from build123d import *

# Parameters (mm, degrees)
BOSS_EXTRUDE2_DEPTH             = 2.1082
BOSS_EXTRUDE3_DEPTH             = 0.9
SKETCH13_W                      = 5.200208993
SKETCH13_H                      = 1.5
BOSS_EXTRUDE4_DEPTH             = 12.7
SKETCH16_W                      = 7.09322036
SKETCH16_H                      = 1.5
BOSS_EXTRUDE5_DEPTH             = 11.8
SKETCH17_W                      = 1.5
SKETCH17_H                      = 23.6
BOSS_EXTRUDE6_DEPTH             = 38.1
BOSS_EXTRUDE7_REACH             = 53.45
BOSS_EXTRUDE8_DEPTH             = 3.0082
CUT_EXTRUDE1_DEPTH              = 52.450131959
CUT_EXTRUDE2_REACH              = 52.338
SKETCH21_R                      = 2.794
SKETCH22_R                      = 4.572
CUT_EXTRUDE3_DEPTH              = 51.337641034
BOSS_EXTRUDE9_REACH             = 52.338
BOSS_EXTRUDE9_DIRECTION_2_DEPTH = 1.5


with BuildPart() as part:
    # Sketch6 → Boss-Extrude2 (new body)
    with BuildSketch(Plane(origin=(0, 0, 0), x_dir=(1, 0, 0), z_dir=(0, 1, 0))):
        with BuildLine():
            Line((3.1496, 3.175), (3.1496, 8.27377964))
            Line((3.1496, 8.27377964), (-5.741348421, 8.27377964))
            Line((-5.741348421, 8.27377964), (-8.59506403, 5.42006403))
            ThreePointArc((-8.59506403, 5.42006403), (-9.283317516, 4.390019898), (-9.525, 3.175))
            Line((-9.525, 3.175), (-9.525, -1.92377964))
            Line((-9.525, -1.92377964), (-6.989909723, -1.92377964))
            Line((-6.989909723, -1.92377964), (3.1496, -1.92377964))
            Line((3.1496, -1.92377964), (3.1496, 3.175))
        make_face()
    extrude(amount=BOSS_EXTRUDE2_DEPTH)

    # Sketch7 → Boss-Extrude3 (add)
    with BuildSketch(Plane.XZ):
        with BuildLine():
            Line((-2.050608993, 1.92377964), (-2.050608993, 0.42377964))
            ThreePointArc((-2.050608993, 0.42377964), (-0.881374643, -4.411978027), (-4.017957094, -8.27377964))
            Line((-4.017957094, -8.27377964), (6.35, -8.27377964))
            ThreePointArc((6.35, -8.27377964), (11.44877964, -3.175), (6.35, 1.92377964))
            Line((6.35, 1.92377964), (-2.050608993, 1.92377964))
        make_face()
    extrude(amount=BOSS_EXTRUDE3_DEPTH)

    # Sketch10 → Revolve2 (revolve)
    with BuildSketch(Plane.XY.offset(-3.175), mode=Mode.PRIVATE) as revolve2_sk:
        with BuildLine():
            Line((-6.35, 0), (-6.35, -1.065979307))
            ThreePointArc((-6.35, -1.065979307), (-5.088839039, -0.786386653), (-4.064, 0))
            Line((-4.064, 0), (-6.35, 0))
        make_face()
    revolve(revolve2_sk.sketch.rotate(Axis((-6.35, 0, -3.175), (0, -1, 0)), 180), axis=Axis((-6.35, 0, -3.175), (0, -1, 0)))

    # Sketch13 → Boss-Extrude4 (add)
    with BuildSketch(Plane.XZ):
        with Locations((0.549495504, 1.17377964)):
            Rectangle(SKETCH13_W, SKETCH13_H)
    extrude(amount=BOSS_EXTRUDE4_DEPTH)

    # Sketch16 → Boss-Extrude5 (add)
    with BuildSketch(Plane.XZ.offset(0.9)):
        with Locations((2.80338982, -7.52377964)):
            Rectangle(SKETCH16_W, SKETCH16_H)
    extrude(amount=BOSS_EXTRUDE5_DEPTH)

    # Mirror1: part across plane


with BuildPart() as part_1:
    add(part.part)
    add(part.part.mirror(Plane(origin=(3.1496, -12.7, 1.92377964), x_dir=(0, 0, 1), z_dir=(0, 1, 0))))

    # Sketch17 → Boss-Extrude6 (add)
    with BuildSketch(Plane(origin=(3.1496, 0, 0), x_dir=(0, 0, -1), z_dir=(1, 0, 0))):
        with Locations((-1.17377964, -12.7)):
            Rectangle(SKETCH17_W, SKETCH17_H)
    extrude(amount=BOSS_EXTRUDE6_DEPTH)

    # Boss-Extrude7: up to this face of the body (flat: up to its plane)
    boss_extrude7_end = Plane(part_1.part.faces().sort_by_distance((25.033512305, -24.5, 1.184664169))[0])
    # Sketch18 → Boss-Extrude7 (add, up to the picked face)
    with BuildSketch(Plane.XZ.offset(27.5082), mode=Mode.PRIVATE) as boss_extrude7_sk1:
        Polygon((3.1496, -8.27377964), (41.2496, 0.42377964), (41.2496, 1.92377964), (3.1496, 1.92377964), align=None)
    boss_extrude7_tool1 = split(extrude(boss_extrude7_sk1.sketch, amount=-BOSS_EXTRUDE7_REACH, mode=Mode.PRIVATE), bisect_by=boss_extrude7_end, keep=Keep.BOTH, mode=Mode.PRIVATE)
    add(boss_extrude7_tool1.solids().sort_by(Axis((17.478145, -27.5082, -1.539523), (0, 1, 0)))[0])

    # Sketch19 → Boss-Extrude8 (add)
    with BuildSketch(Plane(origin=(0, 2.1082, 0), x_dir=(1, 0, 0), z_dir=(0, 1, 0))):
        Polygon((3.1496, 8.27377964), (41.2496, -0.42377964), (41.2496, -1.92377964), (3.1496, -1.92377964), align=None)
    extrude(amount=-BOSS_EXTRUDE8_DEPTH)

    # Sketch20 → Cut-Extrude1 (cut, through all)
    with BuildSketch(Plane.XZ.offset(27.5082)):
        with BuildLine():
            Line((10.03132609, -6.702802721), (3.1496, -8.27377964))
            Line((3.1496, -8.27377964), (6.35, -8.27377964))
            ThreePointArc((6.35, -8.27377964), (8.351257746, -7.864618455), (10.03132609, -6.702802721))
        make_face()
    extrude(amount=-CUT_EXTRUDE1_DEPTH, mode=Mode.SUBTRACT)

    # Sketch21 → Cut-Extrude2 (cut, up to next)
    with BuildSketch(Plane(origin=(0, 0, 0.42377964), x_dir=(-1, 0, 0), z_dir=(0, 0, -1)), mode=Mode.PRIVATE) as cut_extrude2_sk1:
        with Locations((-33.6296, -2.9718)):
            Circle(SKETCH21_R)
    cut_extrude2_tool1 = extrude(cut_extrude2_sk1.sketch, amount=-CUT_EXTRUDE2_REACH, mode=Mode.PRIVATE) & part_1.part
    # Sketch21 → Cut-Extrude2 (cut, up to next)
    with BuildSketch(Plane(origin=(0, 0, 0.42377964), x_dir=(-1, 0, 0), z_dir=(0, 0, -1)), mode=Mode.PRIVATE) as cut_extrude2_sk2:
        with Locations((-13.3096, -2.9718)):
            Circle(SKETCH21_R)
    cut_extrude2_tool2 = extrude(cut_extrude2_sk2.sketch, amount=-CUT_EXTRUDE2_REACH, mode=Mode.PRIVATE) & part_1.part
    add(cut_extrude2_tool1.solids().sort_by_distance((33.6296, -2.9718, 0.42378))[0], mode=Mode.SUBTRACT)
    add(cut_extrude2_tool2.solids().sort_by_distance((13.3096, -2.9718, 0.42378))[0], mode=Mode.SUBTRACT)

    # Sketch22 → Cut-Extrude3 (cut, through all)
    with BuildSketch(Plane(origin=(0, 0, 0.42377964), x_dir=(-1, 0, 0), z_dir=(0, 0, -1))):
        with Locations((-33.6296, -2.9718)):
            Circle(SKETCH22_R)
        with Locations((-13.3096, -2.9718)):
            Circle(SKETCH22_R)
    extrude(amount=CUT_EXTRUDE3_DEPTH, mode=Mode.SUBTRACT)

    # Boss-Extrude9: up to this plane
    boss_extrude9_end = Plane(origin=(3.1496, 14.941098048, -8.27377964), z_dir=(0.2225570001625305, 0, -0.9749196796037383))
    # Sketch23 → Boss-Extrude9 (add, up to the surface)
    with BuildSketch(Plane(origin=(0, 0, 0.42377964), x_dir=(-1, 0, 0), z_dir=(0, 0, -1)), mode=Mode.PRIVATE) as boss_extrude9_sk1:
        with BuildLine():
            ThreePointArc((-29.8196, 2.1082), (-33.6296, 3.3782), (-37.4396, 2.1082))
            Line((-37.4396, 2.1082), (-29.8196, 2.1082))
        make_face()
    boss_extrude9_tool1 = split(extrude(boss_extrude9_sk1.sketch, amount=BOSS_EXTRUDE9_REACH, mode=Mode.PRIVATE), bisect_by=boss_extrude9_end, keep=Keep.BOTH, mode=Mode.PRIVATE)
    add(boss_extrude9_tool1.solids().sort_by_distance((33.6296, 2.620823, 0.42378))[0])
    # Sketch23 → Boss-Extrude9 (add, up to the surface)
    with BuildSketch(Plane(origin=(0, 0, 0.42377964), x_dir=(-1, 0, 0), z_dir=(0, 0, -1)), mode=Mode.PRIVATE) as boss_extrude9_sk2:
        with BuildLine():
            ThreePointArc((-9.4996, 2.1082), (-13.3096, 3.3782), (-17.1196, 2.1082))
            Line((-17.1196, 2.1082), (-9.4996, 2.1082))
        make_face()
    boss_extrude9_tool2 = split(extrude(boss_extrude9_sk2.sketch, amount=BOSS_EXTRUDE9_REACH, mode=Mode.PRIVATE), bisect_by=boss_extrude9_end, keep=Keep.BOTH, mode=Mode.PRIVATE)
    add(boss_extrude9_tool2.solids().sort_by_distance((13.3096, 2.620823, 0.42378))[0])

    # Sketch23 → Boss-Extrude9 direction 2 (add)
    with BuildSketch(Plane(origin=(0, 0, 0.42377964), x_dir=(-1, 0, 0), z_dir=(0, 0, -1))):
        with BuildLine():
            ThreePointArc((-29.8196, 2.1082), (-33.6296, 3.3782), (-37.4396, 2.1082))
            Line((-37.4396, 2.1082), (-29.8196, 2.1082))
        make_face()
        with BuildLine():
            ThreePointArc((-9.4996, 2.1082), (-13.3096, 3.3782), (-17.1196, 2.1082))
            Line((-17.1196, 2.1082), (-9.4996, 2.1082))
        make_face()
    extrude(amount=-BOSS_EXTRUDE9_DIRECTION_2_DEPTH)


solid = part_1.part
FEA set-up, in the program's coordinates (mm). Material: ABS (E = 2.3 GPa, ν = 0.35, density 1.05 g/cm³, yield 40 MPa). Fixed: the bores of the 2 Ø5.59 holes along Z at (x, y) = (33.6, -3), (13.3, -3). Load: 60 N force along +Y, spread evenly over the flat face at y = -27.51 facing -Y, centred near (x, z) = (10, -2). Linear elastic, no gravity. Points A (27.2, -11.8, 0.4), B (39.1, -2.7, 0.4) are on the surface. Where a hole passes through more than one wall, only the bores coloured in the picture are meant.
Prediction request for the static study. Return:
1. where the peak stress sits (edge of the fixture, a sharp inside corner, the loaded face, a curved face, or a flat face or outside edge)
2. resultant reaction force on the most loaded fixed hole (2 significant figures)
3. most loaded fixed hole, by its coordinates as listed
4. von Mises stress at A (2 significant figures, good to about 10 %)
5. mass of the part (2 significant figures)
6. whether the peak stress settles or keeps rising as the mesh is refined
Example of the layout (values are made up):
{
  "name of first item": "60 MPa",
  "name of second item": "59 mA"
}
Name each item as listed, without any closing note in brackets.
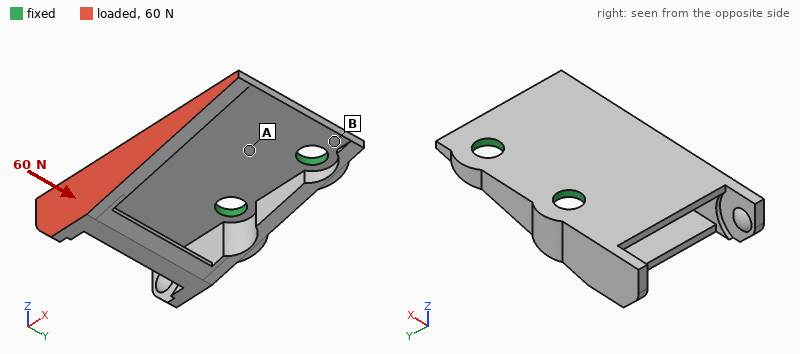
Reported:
{
  "where the peak stress sits": "edge of the fixture",
  "resultant reaction force on the most loaded fixed hole": "61 N",
  "most loaded fixed hole, by its coordinates as listed": "(13.3, -3)",
  "von Mises stress at A": "3.5 MPa",
  "mass of the part": "3.8 g",
  "whether the peak stress settles or keeps rising as the mesh is refined": "keeps rising"
}
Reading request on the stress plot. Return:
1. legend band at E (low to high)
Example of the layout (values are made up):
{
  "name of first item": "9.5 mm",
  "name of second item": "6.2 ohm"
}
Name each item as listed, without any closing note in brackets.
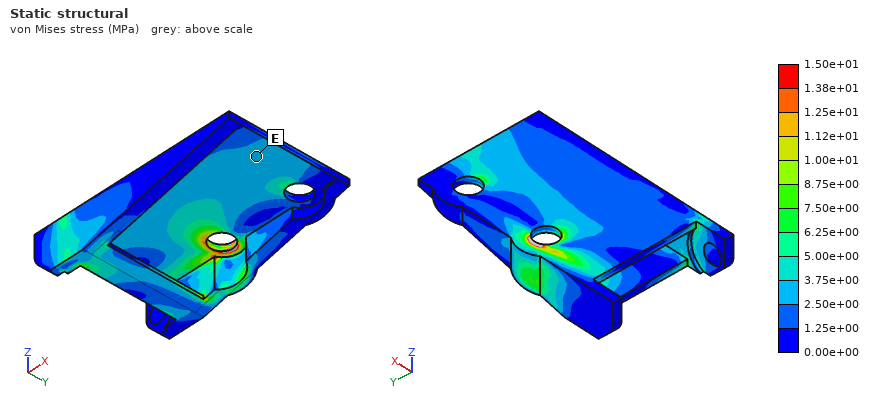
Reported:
{
  "legend band at E": "2.50e+00 to 3.75e+00 MPa"
}
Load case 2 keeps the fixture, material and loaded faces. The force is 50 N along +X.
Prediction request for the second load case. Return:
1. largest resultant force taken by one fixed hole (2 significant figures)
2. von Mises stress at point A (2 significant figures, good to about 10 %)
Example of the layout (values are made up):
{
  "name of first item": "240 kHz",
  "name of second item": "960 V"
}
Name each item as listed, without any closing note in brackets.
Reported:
{
  "largest resultant force taken by one fixed hole": "56 N",
  "von Mises stress at point A": "5.3 MPa"
}
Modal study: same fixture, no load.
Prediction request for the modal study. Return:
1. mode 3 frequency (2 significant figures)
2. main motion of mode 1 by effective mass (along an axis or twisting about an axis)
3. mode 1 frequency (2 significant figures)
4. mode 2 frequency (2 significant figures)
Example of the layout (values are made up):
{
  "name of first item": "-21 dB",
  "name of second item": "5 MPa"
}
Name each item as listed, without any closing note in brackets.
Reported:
{
  "mode 3 frequency": "2000 Hz",
  "main motion of mode 1 by effective mass": "along Z",
  "mode 1 frequency": "500 Hz",
  "mode 2 frequency": "870 Hz"
}
